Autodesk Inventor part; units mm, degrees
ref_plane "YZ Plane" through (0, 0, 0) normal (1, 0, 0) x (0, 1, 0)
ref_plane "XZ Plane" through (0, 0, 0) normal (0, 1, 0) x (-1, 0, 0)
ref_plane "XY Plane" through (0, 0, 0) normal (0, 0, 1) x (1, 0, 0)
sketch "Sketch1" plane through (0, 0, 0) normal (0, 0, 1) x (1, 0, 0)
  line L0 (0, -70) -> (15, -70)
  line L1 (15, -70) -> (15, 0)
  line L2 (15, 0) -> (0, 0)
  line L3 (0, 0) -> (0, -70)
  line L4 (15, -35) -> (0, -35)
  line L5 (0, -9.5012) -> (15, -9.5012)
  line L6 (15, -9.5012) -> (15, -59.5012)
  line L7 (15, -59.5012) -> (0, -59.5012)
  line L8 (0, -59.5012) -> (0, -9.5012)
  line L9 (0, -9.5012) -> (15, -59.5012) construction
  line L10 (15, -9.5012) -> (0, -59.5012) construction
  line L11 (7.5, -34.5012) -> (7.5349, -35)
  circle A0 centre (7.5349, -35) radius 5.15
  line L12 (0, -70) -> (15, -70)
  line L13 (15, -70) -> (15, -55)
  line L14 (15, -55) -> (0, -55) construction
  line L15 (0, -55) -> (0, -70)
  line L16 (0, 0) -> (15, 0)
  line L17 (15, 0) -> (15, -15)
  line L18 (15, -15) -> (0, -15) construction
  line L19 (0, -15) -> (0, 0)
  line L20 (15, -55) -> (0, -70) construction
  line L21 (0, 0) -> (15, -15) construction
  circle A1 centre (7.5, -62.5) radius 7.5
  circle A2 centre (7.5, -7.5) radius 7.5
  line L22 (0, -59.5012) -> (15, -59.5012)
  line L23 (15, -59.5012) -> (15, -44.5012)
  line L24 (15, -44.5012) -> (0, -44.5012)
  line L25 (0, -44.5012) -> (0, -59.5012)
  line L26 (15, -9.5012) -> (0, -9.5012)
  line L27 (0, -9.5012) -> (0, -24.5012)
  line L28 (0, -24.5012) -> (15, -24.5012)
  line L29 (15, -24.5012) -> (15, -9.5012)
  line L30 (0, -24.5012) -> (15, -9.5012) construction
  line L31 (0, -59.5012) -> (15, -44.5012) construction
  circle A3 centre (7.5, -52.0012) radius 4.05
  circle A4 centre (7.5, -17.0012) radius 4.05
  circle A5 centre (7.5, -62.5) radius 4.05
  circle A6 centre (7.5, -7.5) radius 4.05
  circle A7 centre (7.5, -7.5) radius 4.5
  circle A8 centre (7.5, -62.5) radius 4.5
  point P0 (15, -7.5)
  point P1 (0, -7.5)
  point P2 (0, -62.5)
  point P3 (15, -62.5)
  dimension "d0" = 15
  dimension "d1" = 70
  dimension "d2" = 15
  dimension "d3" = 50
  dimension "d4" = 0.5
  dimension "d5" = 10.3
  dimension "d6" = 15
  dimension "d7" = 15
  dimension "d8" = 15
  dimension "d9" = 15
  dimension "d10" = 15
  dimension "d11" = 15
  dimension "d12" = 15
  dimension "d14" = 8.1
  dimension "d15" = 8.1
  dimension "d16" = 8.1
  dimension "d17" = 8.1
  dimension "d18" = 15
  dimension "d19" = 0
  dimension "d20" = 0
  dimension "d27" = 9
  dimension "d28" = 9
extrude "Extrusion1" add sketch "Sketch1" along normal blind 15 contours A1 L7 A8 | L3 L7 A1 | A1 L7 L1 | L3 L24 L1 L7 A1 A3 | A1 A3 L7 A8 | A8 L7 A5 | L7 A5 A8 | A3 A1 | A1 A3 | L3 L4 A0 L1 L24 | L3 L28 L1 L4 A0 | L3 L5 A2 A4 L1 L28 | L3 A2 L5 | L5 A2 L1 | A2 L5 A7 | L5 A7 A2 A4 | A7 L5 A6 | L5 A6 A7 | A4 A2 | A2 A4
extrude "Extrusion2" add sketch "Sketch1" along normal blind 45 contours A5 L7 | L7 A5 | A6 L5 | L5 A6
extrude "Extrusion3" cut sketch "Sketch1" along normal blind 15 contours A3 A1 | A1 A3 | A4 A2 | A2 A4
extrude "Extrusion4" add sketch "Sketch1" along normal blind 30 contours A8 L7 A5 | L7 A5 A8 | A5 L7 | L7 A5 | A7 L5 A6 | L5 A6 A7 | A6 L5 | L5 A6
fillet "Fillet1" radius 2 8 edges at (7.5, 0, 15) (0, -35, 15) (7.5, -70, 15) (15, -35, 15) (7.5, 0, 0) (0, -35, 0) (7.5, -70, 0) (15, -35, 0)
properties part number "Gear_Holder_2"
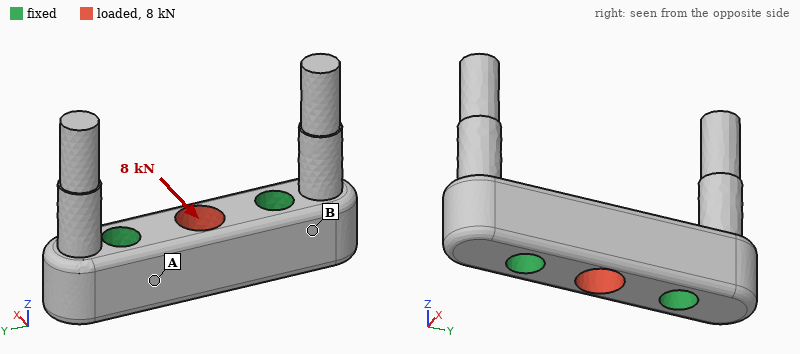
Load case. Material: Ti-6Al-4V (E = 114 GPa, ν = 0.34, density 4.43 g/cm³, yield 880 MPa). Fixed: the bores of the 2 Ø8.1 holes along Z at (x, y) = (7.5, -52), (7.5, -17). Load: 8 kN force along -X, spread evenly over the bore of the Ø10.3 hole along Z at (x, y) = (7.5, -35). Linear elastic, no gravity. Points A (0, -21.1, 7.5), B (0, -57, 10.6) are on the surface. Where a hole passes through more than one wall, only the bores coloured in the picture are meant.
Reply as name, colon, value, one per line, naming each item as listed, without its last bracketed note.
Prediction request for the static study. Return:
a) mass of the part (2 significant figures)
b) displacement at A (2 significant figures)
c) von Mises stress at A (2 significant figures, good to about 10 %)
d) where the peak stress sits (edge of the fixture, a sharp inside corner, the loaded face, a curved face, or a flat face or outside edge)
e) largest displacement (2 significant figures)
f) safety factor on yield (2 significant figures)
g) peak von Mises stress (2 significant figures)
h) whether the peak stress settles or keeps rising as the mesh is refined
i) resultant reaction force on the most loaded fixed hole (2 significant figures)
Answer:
mass of the part: 68 g
displacement at A: 2.5 µm
von Mises stress at A: 33 MPa
where the peak stress sits: a curved face
largest displacement: 12 µm
safety factor on yield: 8.9
peak von Mises stress: 99 MPa
whether the peak stress settles or keeps rising as the mesh is refined: settles
resultant reaction force on the most loaded fixed hole: 4.1 kN
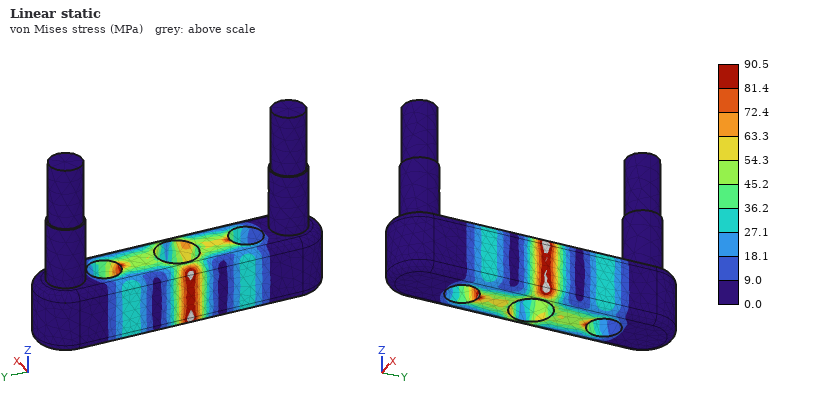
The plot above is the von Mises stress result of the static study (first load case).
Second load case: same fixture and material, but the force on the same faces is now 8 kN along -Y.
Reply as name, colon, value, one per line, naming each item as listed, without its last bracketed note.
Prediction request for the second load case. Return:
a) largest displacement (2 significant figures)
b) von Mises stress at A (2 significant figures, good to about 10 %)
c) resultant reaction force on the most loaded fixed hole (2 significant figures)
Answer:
largest displacement: 2.6 µm
von Mises stress at A: 9.8 MPa
resultant reaction force on the most loaded fixed hole: 4.1 kN
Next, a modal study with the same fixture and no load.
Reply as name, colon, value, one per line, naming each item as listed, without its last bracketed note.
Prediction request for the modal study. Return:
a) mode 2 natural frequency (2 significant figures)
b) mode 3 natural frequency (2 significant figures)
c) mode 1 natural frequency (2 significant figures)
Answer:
mode 2 natural frequency: 6200 Hz
mode 3 natural frequency: 6200 Hz
mode 1 natural frequency: 6100 Hz
